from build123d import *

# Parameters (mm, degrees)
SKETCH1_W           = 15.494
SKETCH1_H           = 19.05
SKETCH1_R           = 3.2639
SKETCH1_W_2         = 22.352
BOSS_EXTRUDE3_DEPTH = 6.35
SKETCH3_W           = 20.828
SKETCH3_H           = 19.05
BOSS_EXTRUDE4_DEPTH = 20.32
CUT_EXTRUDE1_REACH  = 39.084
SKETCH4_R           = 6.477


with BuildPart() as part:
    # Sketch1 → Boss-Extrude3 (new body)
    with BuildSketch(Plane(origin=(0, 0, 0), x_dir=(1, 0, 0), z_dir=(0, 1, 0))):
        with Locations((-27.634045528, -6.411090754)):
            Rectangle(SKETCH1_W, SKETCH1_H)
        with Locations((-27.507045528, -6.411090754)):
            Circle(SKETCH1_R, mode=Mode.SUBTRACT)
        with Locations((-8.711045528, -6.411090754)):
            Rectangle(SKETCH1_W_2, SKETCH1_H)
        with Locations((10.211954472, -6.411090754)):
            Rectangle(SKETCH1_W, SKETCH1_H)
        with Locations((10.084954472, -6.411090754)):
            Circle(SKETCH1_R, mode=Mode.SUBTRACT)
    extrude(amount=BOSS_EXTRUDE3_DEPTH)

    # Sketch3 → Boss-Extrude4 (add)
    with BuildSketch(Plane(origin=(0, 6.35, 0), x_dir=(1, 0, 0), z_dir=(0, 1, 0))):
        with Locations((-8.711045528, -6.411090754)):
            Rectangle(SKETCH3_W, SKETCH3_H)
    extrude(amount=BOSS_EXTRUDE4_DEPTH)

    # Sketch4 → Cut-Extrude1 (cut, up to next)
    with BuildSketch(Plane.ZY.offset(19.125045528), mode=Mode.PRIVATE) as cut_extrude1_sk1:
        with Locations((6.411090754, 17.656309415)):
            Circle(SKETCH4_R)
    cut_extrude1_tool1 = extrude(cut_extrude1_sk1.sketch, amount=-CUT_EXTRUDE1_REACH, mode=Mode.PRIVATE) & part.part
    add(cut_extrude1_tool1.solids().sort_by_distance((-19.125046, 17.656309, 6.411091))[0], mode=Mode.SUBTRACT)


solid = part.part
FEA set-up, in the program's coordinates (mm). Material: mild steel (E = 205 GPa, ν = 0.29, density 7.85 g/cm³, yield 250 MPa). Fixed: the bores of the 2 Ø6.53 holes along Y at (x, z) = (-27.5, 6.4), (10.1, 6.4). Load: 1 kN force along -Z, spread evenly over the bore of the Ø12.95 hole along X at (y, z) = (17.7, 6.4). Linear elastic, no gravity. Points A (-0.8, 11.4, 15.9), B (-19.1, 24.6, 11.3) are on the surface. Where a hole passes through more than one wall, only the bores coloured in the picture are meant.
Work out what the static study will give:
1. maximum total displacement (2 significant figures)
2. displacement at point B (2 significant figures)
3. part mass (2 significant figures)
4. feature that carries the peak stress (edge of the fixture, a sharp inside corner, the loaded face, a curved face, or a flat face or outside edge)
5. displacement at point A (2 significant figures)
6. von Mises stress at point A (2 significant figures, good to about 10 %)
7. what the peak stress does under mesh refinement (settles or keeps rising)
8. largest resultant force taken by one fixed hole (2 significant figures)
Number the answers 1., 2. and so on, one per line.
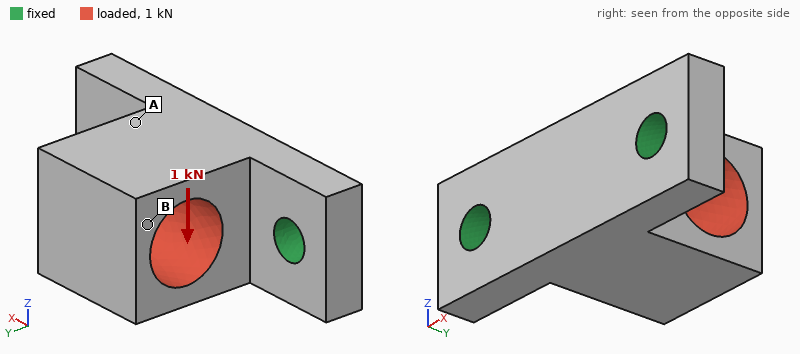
1. 17 µm
2. 15 µm
3. 89 g
4. edge of the fixture
5. 7.2 µm
6. 21 MPa
7. keeps rising
8. 500 N
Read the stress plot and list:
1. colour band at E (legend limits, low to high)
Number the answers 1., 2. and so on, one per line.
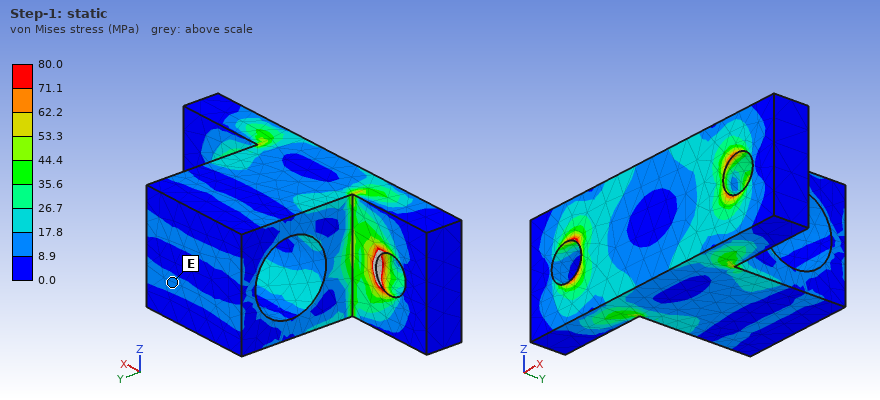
1. 8.9 to 17.8 MPa
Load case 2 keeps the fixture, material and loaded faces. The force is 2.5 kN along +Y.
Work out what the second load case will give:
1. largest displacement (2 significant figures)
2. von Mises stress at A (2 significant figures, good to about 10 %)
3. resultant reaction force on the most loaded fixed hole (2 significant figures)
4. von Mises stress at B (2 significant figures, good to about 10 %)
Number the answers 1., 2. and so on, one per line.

1. 5.5 µm
2. 18 MPa
3. 1.3 kN
4. 8.3 MPa
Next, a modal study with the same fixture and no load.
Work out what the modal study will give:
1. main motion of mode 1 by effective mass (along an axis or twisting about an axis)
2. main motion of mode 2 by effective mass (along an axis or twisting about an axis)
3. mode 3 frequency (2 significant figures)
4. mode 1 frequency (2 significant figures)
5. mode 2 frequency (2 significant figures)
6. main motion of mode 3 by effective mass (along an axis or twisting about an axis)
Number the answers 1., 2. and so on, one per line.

1. along Z
2. along X
3. 17 kHz
4. 7200 Hz
5. 15 kHz
6. along Y
